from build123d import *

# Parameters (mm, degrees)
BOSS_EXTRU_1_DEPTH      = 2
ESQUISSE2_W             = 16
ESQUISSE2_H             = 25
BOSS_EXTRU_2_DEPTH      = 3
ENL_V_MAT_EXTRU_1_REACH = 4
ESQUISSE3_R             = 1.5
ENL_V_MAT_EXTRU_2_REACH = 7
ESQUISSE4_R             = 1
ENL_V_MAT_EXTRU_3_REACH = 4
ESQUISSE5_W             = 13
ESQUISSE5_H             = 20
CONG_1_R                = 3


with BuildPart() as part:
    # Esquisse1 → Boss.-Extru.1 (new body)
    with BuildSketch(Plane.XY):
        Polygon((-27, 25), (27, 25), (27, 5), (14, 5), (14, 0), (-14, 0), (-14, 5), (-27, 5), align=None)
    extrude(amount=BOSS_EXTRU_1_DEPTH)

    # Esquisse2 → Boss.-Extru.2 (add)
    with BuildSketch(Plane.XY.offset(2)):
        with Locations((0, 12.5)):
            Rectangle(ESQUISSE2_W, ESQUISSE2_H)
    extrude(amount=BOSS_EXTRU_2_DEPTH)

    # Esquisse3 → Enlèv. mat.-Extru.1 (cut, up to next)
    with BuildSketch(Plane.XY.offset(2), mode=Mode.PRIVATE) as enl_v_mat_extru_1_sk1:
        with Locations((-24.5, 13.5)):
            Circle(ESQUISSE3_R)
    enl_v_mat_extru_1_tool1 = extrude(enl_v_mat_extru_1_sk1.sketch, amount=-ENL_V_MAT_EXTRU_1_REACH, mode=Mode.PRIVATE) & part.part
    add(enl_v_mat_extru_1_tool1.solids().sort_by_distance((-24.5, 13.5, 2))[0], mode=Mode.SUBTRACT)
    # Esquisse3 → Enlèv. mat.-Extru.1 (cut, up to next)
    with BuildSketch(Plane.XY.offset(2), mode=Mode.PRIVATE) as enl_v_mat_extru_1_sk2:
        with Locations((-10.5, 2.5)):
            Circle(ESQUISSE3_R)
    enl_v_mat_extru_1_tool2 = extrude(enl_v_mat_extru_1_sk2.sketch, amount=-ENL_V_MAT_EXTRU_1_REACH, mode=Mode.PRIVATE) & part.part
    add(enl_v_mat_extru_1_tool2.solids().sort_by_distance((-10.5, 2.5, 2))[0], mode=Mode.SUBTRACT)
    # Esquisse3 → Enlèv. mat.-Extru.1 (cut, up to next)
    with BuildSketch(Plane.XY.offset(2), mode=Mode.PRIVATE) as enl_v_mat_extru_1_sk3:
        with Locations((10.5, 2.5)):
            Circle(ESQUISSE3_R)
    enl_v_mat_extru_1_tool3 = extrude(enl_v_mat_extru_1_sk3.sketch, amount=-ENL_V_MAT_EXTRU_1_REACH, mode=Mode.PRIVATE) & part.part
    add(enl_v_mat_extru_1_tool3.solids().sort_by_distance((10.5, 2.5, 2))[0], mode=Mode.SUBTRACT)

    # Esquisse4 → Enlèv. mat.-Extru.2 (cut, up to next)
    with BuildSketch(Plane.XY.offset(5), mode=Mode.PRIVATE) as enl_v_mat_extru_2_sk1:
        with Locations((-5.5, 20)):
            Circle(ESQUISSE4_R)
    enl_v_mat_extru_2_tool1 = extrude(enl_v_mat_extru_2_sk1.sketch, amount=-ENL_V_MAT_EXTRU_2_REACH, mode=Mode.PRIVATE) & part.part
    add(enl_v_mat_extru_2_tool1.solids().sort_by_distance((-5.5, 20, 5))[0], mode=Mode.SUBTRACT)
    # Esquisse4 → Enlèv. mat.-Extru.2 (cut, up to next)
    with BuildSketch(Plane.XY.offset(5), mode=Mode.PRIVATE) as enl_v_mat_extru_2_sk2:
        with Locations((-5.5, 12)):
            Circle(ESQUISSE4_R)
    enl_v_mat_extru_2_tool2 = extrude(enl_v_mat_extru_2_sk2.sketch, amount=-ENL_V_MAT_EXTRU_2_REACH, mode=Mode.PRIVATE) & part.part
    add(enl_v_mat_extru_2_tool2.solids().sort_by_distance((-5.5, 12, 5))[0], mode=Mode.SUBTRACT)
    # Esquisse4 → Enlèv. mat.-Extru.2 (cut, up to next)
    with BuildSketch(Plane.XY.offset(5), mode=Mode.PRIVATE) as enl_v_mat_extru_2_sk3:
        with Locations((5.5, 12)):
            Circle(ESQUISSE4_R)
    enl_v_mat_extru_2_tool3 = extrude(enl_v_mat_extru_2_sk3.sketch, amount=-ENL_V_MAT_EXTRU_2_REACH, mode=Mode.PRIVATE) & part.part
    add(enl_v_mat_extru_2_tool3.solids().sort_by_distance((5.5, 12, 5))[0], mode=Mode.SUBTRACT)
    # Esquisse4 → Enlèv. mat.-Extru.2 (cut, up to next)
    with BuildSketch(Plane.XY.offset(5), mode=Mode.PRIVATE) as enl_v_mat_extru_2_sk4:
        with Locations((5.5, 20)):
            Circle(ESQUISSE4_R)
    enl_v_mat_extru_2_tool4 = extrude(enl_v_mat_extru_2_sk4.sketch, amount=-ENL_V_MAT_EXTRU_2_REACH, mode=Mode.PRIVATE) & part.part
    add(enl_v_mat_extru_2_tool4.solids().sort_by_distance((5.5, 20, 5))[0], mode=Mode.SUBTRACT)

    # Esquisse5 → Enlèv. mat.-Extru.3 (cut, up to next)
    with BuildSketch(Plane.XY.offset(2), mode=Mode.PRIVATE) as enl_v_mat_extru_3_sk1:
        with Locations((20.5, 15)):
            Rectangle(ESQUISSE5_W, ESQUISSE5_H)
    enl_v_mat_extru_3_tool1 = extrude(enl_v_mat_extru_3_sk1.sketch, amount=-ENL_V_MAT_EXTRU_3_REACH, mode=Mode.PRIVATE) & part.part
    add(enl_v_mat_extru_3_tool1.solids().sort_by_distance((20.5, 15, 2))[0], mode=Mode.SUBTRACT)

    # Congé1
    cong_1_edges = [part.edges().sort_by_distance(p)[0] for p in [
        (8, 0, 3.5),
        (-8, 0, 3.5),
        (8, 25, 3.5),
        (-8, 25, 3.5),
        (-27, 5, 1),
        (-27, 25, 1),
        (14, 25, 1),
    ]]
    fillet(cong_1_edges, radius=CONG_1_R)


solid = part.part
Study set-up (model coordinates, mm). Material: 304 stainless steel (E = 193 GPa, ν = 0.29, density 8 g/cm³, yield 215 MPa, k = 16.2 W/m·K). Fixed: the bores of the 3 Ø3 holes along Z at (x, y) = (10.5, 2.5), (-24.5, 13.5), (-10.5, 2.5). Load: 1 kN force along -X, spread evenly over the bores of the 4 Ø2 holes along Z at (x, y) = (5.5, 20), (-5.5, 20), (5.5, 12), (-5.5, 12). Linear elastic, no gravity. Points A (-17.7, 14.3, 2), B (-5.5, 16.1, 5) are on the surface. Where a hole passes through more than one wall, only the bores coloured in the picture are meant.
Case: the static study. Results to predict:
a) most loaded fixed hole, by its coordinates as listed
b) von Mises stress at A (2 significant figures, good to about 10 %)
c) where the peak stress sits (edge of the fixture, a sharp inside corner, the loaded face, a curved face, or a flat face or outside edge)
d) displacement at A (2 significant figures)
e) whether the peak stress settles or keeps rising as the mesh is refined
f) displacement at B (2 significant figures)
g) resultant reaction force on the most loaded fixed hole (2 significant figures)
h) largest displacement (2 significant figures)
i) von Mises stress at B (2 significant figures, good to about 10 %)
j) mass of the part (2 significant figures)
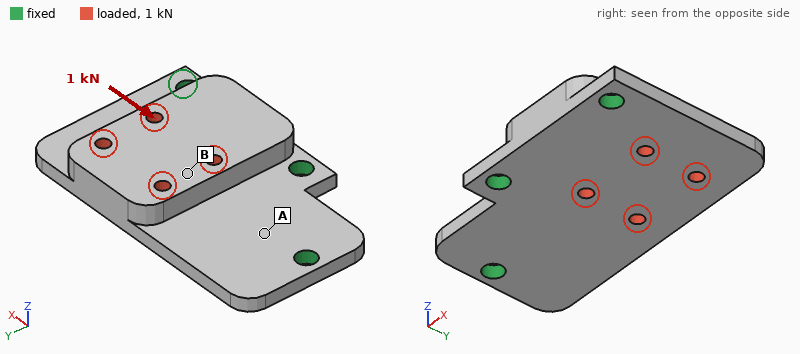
(10.5, 2.5)
20 MPa
edge of the fixture
0.68 µm
keeps rising
2.2 µm
480 N
3.9 µm
9.5 MPa
24 g
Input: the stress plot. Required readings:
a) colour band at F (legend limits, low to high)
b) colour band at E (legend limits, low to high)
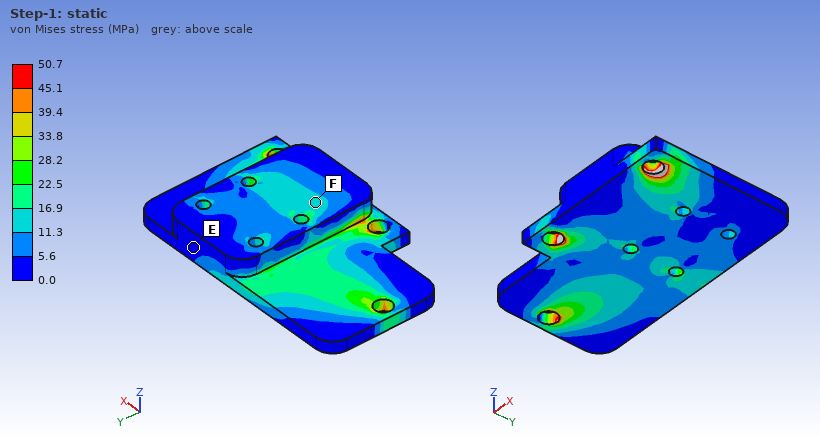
11.3 to 16.9 MPa
0.0 to 5.6 MPa
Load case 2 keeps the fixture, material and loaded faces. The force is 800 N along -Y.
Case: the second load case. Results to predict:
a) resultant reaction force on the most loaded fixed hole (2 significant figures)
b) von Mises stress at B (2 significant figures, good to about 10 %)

410 N
6.6 MPa
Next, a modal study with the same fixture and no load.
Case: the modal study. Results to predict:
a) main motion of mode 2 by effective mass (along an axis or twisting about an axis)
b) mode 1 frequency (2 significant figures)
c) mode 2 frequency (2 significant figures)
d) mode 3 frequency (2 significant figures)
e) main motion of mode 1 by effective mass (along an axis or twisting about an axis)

twisting about Y
4100 Hz
13 kHz
19 kHz
along Z
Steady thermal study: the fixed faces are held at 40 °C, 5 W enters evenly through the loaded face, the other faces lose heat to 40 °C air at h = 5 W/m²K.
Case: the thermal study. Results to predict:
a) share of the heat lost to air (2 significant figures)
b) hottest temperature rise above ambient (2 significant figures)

6.1 %
51 K
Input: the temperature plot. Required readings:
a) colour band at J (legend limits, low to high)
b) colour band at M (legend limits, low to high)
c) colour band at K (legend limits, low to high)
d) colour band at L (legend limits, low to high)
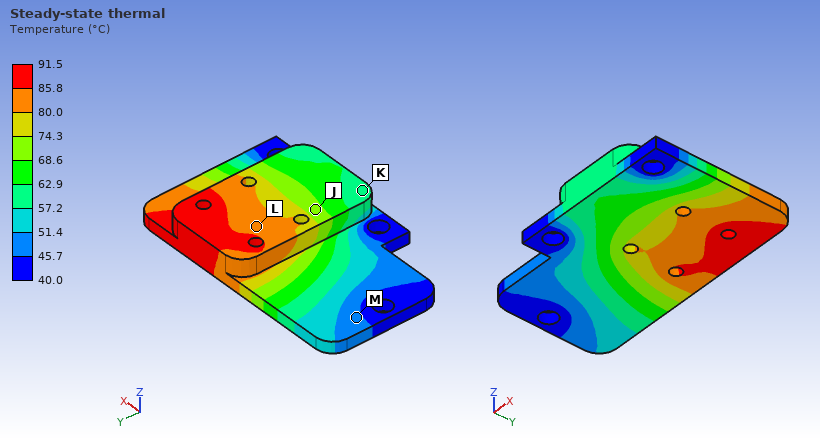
68.6 to 74.3 °C
45.7 to 51.4 °C
57.2 to 62.9 °C
80.0 to 85.8 °C
